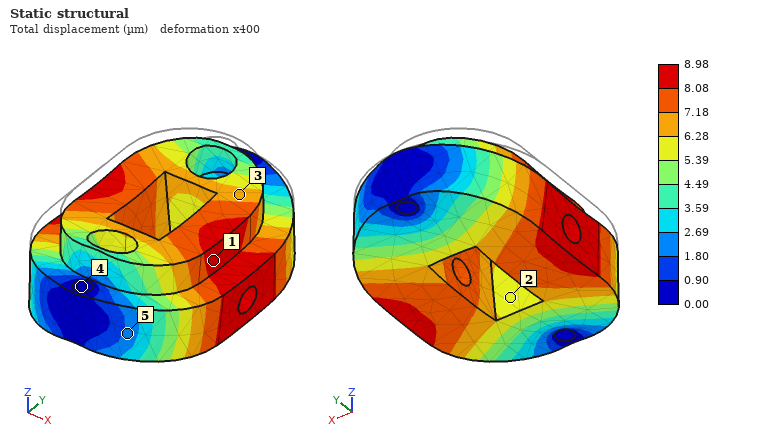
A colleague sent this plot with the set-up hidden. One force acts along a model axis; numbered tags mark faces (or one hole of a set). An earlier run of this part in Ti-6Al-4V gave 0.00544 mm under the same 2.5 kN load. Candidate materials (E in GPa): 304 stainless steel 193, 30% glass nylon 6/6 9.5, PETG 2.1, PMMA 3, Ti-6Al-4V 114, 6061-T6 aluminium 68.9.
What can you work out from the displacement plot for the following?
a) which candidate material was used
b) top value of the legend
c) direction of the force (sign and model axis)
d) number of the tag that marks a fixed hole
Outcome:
6061-T6 aluminium
8.98 µm
-Z
4
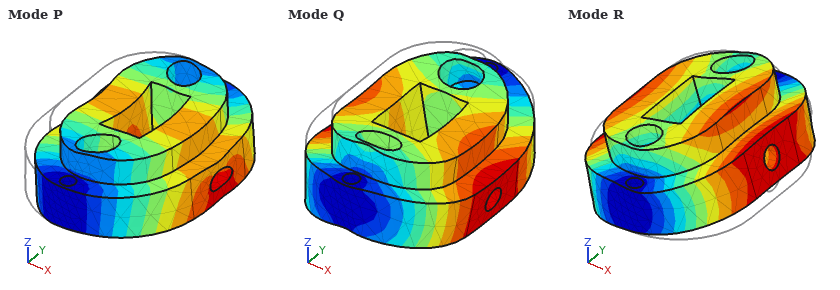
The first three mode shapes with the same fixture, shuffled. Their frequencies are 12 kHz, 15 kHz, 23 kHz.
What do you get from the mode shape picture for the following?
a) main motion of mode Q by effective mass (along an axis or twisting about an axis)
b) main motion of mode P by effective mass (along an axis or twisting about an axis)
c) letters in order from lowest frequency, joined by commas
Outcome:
along Z
along X
R, Q, P
